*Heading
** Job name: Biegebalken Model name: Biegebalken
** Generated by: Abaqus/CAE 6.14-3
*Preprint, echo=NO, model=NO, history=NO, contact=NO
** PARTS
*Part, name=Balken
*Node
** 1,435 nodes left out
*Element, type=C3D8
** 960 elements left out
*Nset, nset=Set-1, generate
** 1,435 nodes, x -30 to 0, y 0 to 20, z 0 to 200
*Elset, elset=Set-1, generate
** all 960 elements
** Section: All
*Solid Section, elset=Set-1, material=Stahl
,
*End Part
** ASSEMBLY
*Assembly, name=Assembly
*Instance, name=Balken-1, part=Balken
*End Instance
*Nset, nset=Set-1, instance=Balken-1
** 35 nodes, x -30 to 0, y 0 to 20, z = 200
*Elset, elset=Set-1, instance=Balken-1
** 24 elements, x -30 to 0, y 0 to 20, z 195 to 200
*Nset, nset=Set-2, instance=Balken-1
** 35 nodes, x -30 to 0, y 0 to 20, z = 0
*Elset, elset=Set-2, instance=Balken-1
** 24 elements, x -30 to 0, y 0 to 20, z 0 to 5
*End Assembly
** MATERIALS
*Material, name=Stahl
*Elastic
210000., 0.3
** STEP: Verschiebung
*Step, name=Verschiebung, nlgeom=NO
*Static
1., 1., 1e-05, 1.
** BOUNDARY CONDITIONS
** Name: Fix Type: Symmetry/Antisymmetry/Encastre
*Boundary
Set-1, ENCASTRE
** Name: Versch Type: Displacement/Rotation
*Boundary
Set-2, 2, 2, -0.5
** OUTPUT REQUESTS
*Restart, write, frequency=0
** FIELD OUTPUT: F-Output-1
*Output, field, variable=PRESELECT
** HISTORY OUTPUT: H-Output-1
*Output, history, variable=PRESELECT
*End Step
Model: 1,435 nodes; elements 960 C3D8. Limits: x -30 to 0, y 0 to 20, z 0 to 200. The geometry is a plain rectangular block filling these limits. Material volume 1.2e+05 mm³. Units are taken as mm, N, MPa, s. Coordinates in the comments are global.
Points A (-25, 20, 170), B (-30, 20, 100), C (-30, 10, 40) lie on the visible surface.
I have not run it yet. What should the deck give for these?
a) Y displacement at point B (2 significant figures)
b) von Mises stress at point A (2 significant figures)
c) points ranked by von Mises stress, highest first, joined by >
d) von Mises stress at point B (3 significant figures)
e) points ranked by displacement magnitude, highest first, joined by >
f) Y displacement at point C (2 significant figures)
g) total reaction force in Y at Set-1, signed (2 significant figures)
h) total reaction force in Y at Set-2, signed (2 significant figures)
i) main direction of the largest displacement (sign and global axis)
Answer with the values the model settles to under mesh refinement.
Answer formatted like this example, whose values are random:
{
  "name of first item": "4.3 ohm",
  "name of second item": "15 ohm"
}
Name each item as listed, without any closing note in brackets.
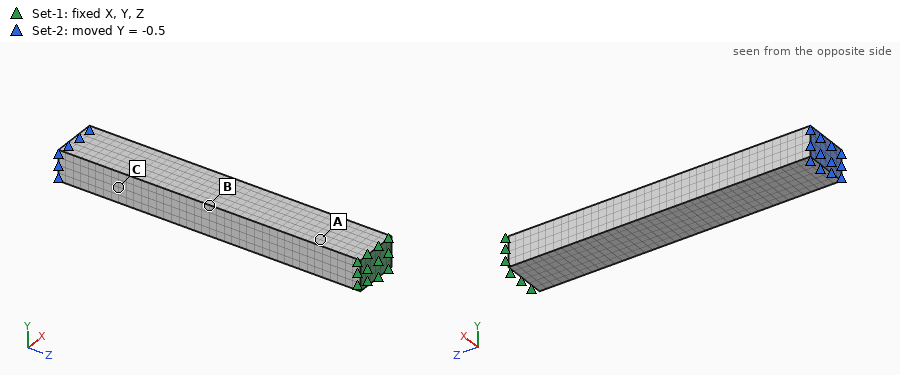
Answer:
{
  "Y displacement at point B": "-0.16 mm",
  "von Mises stress at point A": "67 MPa",
  "points ranked by von Mises stress, highest first, joined by >": "A > B > C",
  "von Mises stress at point B": "39.5 MPa",
  "points ranked by displacement magnitude, highest first, joined by >": "C > B > A",
  "Y displacement at point C": "-0.35 mm",
  "total reaction force in Y at Set-1, signed": "790 N",
  "total reaction force in Y at Set-2, signed": "-790 N",
  "main direction of the largest displacement": "-Y"
}
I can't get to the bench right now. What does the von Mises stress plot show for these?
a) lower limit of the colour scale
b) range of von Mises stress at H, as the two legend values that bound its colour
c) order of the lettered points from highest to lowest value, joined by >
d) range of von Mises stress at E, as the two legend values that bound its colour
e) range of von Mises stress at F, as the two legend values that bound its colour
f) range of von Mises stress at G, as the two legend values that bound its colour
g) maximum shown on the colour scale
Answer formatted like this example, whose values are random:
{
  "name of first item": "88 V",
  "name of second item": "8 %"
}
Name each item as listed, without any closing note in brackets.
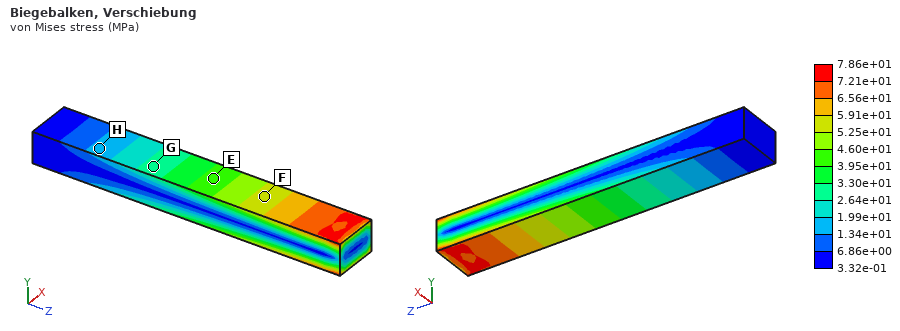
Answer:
{
  "lower limit of the colour scale": "3.32e-01 MPa",
  "range of von Mises stress at H, as the two legend values that bound its colour": "1.34e+01 to 1.99e+01 MPa",
  "order of the lettered points from highest to lowest value, joined by >": "F > E > G > H",
  "range of von Mises stress at E, as the two legend values that bound its colour": "3.95e+01 to 4.60e+01 MPa",
  "range of von Mises stress at F, as the two legend values that bound its colour": "5.25e+01 to 5.91e+01 MPa",
  "range of von Mises stress at G, as the two legend values that bound its colour": "2.64e+01 to 3.30e+01 MPa",
  "maximum shown on the colour scale": "7.86e+01 MPa"
}
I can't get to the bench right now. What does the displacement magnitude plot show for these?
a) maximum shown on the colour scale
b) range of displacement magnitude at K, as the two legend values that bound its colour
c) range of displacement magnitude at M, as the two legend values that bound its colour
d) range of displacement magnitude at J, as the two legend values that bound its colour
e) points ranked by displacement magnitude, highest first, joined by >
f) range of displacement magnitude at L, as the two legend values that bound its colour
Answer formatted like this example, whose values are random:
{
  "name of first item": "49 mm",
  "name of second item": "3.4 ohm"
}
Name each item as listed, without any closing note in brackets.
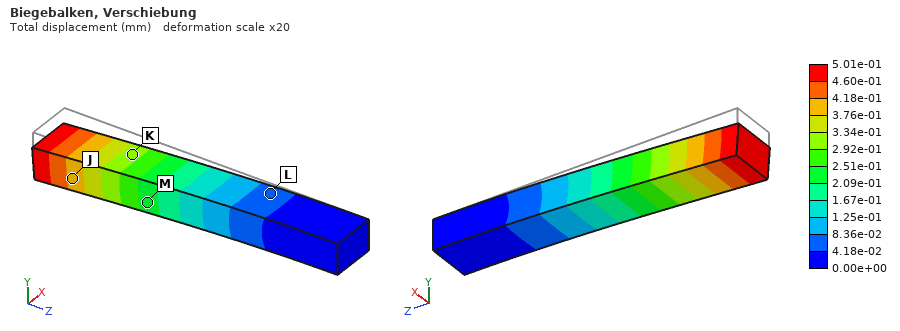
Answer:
{
  "maximum shown on the colour scale": "5.01e-01 mm",
  "range of displacement magnitude at K, as the two legend values that bound its colour": "2.92e-01 to 3.34e-01 mm",
  "range of displacement magnitude at M, as the two legend values that bound its colour": "2.09e-01 to 2.51e-01 mm",
  "range of displacement magnitude at J, as the two legend values that bound its colour": "3.76e-01 to 4.18e-01 mm",
  "points ranked by displacement magnitude, highest first, joined by >": "J > K > M > L",
  "range of displacement magnitude at L, as the two legend values that bound its colour": "4.18e-02 to 8.36e-02 mm"
}
